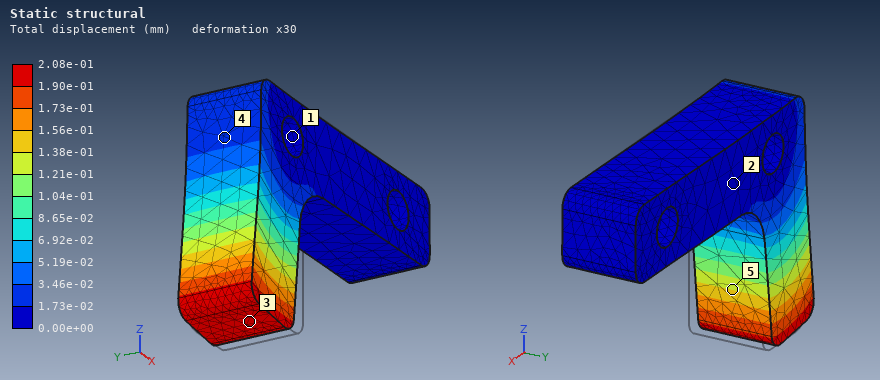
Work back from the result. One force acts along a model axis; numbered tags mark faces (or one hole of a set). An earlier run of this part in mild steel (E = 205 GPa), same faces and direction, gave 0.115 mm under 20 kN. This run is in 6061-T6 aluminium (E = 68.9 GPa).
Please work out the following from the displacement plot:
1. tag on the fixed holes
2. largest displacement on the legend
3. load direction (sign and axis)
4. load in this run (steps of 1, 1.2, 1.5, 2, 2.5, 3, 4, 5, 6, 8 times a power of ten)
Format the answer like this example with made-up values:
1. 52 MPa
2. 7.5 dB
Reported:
1. 1
2. 2.08e-01 mm
3. -X
4. 12 kN
